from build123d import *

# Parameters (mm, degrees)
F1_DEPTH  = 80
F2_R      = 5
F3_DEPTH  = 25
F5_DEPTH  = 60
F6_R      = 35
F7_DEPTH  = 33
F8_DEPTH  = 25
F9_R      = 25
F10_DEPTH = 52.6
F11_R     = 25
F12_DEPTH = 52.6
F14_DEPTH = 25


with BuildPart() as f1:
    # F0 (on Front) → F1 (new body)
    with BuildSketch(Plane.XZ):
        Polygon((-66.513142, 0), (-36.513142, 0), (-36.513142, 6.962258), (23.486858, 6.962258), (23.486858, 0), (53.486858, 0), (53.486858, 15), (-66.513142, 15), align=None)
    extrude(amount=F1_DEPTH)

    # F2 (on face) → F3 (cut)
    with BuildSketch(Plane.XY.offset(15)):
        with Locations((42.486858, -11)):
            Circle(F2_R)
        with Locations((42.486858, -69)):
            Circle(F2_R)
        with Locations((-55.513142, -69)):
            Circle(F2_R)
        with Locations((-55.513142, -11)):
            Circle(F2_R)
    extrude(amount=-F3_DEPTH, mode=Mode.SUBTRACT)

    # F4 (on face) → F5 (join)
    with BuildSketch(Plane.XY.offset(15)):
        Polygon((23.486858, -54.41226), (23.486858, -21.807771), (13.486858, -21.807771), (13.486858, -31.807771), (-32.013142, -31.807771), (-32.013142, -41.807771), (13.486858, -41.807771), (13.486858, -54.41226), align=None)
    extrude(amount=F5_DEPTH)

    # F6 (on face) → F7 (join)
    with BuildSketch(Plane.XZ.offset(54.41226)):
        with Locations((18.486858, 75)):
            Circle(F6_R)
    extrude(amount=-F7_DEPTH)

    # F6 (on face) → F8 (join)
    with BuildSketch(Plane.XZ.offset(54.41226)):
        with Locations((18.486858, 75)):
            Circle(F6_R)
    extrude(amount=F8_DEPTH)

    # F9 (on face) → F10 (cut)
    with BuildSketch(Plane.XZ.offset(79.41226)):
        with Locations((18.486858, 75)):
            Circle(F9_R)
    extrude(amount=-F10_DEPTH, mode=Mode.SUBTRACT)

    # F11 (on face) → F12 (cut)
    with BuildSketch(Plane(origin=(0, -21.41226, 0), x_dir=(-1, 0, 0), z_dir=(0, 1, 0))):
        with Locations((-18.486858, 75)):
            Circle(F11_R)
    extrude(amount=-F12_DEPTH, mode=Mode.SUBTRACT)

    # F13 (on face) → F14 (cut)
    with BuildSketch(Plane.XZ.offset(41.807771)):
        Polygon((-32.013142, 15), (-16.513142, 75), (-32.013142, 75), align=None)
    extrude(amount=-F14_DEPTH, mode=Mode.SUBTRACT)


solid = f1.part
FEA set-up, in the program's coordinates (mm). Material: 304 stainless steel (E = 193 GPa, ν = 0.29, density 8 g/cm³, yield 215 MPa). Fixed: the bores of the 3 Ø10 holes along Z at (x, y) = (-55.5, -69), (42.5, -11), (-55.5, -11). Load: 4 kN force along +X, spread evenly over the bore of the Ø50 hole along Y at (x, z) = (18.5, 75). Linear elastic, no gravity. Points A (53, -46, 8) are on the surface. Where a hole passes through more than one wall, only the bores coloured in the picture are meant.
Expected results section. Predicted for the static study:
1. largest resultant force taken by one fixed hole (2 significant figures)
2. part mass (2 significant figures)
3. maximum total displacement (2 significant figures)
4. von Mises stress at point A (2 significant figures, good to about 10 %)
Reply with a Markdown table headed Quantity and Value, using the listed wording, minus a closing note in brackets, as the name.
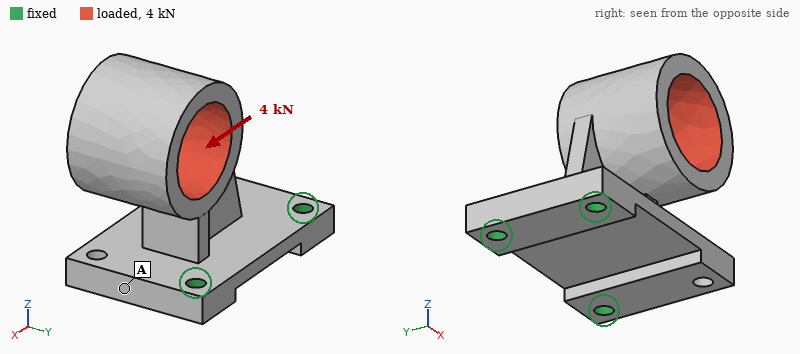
| Quantity | Value |
|---|---|
| largest resultant force taken by one fixed hole | 4.0 kN |
| part mass | 1.9 kg |
| maximum total displacement | 0.11 mm |
| von Mises stress at point A | 8.3 MPa |
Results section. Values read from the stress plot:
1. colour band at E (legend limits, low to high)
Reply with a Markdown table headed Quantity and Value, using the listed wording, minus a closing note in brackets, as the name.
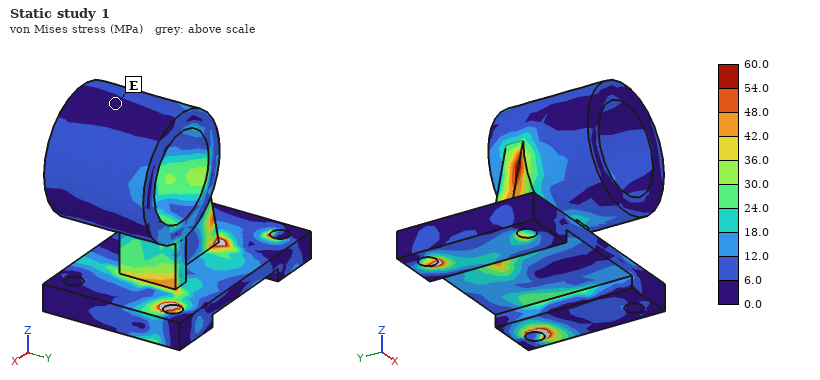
| Quantity | Value |
|---|---|
| colour band at E | 0.0 to 6.0 MPa |
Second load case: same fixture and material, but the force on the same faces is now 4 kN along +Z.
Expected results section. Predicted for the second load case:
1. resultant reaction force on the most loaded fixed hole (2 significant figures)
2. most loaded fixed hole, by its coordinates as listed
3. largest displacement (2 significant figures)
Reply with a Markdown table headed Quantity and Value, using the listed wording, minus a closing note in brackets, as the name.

| Quantity | Value |
|---|---|
| resultant reaction force on the most loaded fixed hole | 3.4 kN |
| most loaded fixed hole, by its coordinates as listed | (42.5, -11) |
| largest displacement | 0.14 mm |
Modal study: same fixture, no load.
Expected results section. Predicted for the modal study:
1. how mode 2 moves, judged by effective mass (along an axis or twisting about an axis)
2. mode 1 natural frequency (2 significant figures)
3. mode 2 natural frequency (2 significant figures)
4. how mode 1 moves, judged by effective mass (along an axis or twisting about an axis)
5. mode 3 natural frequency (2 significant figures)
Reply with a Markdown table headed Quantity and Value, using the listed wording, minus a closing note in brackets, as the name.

| Quantity | Value |
|---|---|
| how mode 2 moves, judged by effective mass | along X |
| mode 1 natural frequency | 640 Hz |
| mode 2 natural frequency | 1200 Hz |
| how mode 1 moves, judged by effective mass | along Y |
| mode 3 natural frequency | 1800 Hz |
